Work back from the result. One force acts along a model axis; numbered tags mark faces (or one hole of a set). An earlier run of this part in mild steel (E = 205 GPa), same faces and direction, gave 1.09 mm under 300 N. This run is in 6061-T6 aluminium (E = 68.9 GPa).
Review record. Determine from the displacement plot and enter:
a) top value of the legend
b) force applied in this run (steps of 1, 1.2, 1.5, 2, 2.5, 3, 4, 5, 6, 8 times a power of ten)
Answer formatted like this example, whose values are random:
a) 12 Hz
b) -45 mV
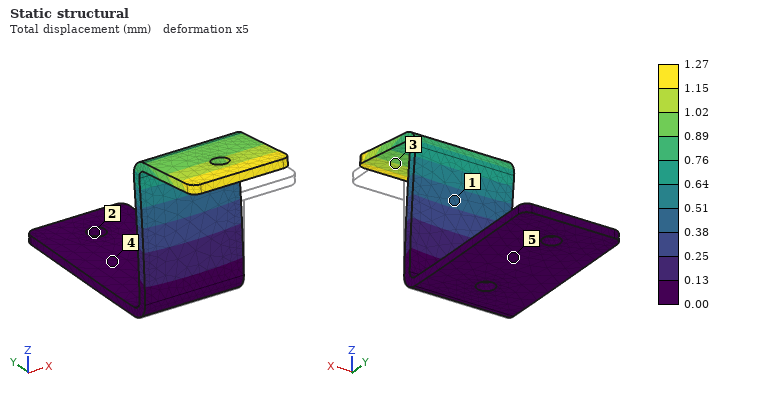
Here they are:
a) 1.27 mm
b) 120 N
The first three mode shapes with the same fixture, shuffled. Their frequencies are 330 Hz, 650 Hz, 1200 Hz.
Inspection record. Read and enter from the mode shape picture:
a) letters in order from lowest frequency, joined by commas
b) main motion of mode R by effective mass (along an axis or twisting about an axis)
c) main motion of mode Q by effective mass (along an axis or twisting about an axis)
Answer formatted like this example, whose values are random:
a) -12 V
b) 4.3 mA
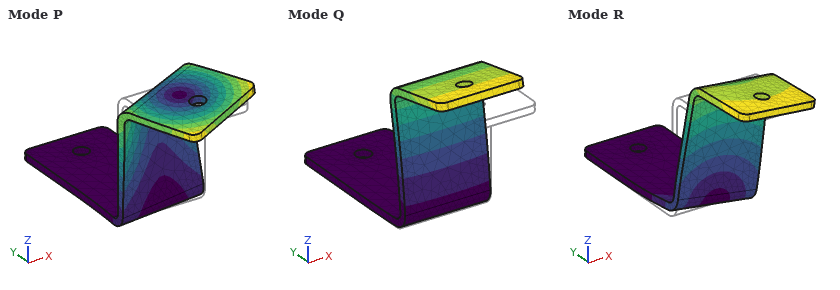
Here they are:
a) Q, R, P
b) along X
c) along Y
